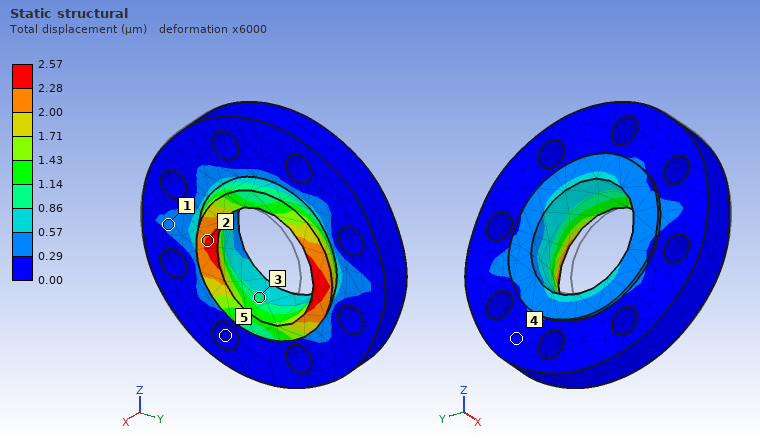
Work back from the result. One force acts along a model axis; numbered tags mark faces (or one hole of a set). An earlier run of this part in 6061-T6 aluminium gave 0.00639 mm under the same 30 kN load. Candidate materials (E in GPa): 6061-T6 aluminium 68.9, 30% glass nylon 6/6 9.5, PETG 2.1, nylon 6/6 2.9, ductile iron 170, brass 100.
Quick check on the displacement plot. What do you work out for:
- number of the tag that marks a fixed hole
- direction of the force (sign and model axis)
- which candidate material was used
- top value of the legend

5
+Y
ductile iron
2.57 µm
